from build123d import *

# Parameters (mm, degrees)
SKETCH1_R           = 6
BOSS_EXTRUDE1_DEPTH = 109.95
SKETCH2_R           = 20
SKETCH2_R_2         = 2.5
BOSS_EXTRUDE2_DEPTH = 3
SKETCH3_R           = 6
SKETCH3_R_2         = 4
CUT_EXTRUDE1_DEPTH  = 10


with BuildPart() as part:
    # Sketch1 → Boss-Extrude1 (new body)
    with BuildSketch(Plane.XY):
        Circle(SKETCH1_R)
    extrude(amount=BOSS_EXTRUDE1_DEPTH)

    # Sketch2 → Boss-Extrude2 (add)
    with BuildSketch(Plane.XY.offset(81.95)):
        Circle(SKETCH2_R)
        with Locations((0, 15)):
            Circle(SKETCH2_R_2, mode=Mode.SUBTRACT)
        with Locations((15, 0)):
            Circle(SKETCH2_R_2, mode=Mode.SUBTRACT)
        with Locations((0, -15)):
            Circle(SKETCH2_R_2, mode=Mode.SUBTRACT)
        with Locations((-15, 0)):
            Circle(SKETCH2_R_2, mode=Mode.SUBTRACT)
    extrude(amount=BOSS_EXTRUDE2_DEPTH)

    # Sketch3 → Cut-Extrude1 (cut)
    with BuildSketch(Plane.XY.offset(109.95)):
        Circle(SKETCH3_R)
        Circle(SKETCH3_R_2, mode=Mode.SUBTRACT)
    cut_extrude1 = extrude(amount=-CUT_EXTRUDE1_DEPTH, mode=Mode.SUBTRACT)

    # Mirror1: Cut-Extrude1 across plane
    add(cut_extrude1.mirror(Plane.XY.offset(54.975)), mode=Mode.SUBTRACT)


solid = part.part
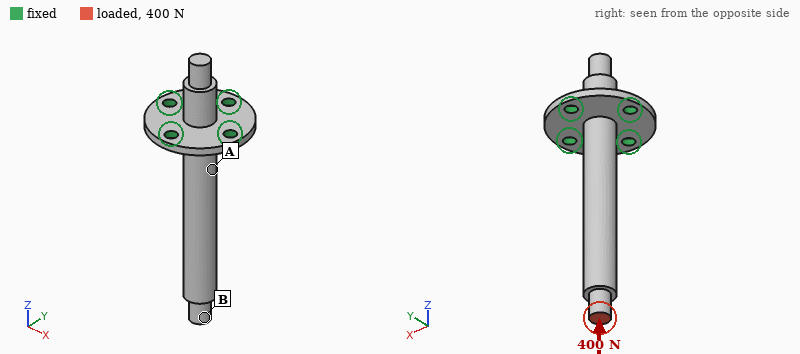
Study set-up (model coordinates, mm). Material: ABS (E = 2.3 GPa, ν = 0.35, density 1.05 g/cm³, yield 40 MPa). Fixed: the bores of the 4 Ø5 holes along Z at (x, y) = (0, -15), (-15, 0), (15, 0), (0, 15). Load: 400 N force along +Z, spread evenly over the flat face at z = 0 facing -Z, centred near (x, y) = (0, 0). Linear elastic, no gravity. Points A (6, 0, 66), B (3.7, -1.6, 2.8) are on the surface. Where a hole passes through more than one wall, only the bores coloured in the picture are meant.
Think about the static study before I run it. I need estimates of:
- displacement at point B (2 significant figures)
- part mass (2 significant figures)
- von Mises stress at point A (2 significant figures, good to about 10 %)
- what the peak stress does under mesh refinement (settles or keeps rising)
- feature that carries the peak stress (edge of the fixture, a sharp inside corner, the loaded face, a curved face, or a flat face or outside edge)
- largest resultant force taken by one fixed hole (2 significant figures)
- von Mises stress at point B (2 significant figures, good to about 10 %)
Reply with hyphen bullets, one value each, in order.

- 0.24 mm
- 15 g
- 3.5 MPa
- keeps rising
- edge of the fixture
- 100 N
- 7.9 MPa
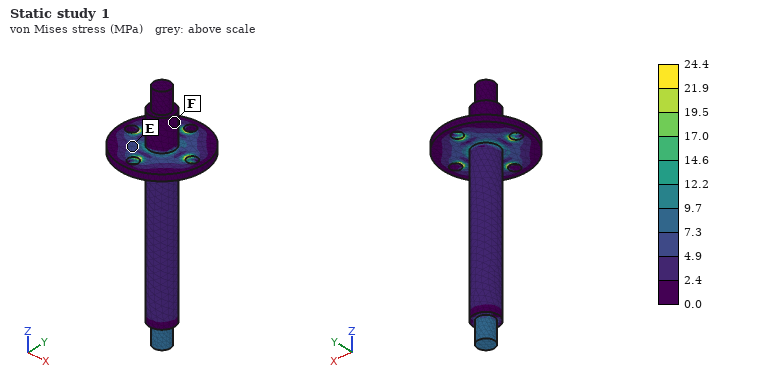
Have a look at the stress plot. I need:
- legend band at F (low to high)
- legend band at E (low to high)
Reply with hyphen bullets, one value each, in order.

- 0.0 to 2.4 MPa
- 4.9 to 7.3 MPa
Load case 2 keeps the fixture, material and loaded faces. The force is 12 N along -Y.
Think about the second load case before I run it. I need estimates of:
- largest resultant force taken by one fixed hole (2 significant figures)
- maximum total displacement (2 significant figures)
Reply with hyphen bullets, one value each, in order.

- 42 N
- 1.4 mm
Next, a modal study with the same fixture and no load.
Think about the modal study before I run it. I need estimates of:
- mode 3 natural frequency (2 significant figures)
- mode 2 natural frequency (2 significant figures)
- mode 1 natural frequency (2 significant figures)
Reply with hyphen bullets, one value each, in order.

- 1900 Hz
- 320 Hz
- 320 Hz
